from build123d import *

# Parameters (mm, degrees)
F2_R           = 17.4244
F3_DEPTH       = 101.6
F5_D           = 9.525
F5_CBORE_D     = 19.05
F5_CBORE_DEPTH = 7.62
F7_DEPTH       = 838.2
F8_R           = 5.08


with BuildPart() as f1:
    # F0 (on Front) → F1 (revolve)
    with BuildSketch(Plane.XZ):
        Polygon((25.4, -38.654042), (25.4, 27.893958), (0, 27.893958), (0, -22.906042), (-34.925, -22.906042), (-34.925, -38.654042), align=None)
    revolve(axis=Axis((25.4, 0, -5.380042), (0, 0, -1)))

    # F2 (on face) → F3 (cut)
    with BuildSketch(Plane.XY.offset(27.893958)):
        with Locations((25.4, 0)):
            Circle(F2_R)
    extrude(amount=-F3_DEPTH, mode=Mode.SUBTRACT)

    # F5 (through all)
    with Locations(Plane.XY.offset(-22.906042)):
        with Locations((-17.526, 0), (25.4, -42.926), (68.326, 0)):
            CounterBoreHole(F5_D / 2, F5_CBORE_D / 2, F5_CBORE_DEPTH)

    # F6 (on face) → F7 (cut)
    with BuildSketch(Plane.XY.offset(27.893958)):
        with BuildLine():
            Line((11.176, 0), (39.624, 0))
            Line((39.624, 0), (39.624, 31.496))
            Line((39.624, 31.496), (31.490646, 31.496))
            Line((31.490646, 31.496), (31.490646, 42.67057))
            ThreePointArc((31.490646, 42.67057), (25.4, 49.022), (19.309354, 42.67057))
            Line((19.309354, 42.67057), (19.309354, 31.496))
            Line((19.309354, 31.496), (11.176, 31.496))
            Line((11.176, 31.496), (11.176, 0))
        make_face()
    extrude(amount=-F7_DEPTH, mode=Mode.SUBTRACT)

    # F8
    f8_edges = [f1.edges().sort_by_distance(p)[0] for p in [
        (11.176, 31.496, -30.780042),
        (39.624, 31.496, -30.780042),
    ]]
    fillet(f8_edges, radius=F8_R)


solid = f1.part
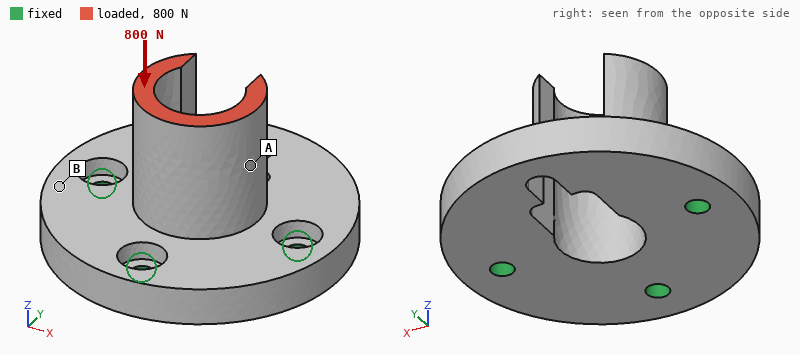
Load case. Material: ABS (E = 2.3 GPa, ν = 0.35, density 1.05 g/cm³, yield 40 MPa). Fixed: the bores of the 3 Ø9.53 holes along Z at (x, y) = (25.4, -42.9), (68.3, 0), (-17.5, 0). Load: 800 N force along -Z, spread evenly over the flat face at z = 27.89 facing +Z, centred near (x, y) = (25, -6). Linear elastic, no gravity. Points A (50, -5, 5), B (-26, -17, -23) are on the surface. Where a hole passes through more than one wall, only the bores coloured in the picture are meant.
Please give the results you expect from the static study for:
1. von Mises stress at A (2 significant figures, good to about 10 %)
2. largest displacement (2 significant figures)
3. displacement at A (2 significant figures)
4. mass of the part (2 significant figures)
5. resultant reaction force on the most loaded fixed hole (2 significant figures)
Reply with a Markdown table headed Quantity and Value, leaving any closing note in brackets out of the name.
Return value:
| Quantity | Value |
|---|---|
| von Mises stress at A | 1.1 MPa |
| largest displacement | 0.15 mm |
| displacement at A | 0.091 mm |
| mass of the part | 200 g |
| resultant reaction force on the most loaded fixed hole | 350 N |
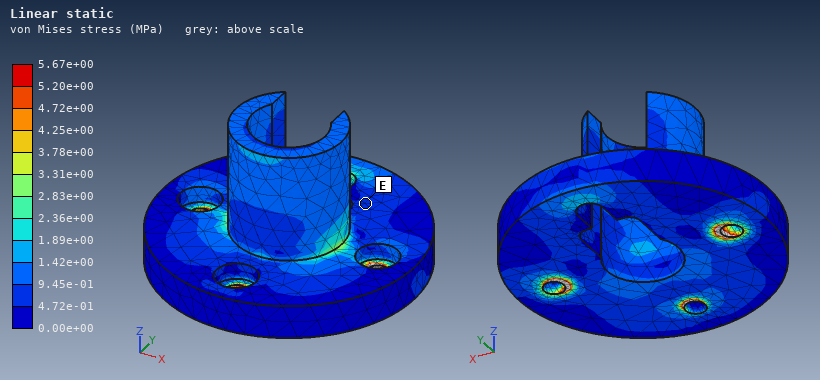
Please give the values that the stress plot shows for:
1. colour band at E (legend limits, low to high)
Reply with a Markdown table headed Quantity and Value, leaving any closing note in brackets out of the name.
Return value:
| Quantity | Value |
|---|---|
| colour band at E | 4.72e-01 to 9.45e-01 MPa |
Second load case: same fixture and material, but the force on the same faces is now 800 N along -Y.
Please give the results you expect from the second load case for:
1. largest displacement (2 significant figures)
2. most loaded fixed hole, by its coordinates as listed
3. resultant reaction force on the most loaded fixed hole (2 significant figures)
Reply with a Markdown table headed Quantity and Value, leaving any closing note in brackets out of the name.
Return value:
| Quantity | Value |
|---|---|
| largest displacement | 0.82 mm |
| most loaded fixed hole, by its coordinates as listed | (25.4, -42.9) |
| resultant reaction force on the most loaded fixed hole | 1.1 kN |
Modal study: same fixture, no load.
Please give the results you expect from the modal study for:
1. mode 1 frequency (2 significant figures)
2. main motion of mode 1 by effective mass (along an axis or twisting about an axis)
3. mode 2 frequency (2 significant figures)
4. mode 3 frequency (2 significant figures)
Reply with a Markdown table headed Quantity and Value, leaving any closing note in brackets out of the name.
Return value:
| Quantity | Value |
|---|---|
| mode 1 frequency | 760 Hz |
| main motion of mode 1 by effective mass | along Z |
| mode 2 frequency | 1100 Hz |
| mode 3 frequency | 1500 Hz |
